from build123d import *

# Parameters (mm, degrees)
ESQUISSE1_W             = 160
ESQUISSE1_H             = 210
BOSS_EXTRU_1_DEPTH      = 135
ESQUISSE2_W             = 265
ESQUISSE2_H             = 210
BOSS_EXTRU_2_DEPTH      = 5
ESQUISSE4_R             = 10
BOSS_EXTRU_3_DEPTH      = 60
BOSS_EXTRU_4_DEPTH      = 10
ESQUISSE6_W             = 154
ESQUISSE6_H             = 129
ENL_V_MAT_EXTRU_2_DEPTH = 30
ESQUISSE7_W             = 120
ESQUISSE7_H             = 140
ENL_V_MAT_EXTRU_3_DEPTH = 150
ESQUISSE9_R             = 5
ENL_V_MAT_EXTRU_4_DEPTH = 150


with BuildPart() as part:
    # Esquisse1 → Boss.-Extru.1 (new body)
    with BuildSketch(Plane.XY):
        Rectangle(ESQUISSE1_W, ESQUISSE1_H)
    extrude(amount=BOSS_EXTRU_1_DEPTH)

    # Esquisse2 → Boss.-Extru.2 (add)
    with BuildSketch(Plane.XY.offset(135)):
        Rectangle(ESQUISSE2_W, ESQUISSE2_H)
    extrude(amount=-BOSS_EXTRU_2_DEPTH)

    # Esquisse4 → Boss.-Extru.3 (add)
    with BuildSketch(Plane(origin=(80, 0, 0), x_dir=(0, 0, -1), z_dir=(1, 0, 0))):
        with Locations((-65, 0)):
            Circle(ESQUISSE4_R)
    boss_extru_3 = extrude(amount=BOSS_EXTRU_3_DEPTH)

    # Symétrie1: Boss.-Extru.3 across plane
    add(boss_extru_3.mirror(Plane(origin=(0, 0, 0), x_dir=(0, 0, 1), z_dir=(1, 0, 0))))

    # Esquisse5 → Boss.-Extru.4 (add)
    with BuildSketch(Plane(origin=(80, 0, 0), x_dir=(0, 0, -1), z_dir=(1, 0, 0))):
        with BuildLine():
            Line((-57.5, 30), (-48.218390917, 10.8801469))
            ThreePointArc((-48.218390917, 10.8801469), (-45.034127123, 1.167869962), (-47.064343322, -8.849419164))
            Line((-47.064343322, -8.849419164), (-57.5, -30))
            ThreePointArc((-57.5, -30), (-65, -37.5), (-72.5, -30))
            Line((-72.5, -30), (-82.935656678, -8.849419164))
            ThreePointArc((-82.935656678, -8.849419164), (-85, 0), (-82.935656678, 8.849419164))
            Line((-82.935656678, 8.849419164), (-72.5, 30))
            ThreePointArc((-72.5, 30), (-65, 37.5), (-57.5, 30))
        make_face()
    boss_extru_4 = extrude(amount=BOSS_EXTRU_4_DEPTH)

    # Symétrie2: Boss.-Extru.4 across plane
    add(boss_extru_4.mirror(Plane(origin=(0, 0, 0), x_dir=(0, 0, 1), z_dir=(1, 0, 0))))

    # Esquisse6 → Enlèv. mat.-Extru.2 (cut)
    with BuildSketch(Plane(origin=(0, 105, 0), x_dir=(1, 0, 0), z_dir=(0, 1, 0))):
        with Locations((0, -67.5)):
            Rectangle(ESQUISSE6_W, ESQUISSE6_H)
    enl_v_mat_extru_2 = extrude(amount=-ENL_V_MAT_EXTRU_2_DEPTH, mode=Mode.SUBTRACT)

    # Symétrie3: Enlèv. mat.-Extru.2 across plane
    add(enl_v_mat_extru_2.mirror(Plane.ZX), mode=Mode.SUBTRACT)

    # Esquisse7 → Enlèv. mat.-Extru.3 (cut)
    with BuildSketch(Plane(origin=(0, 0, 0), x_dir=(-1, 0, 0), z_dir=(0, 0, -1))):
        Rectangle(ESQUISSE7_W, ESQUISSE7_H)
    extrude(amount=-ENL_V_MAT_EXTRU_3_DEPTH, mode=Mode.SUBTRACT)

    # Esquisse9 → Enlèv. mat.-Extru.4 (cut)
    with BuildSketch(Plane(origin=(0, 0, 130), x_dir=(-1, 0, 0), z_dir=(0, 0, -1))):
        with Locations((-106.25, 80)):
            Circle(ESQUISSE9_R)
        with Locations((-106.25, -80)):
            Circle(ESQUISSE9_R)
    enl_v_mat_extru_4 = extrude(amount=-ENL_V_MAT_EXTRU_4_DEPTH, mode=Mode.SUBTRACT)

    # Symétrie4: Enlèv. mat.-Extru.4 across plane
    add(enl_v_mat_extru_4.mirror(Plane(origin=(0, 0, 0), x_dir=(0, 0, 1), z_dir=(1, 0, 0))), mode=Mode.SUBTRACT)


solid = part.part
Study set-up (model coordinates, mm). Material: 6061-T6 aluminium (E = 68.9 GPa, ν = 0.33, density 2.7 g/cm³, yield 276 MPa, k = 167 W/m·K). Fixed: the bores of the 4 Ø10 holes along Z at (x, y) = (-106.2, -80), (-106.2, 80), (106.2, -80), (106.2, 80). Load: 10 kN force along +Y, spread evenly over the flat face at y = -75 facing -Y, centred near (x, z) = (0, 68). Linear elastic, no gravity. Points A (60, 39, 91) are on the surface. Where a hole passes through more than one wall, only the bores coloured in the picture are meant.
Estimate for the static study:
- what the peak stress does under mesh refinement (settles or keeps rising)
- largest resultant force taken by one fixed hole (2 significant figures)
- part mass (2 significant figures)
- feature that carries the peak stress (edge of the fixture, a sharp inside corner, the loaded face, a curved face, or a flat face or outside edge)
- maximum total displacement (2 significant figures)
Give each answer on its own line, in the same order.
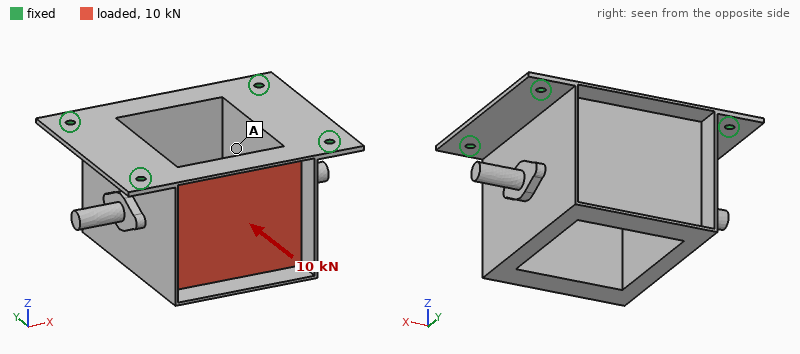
keeps rising
3.7 kN
3.4 kg
edge of the fixture
0.44 mm
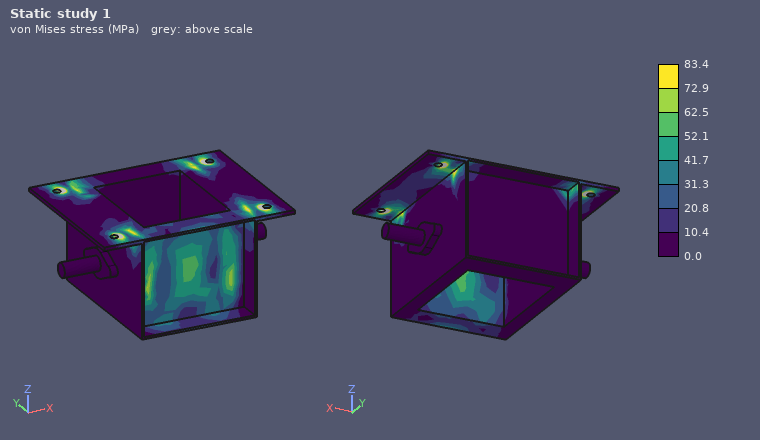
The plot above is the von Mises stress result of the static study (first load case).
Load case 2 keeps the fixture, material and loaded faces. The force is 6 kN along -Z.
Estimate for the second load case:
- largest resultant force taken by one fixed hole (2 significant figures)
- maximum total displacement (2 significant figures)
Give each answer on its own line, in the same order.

3.2 kN
0.27 mm
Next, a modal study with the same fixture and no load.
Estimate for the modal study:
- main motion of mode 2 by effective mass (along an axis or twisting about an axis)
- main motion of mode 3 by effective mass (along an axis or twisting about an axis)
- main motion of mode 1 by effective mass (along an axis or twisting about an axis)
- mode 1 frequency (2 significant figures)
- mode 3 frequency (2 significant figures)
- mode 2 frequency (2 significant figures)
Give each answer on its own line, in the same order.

along X
along Z
along Y
600 Hz
710 Hz
640 Hz
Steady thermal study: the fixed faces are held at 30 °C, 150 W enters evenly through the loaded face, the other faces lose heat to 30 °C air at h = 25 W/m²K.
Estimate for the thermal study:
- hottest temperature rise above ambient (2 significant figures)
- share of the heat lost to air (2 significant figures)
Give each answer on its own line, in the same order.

33 K
58 %
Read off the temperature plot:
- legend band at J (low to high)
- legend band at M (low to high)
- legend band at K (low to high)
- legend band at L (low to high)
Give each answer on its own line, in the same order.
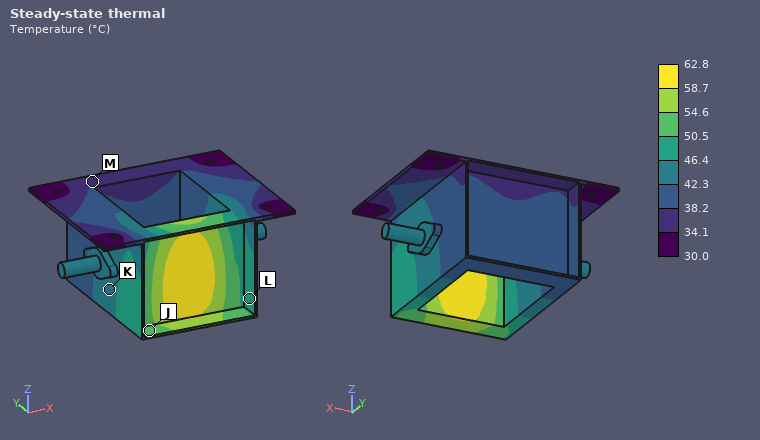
50.5 to 54.6 °C
34.1 to 38.2 °C
42.3 to 46.4 °C
46.4 to 50.5 °C
